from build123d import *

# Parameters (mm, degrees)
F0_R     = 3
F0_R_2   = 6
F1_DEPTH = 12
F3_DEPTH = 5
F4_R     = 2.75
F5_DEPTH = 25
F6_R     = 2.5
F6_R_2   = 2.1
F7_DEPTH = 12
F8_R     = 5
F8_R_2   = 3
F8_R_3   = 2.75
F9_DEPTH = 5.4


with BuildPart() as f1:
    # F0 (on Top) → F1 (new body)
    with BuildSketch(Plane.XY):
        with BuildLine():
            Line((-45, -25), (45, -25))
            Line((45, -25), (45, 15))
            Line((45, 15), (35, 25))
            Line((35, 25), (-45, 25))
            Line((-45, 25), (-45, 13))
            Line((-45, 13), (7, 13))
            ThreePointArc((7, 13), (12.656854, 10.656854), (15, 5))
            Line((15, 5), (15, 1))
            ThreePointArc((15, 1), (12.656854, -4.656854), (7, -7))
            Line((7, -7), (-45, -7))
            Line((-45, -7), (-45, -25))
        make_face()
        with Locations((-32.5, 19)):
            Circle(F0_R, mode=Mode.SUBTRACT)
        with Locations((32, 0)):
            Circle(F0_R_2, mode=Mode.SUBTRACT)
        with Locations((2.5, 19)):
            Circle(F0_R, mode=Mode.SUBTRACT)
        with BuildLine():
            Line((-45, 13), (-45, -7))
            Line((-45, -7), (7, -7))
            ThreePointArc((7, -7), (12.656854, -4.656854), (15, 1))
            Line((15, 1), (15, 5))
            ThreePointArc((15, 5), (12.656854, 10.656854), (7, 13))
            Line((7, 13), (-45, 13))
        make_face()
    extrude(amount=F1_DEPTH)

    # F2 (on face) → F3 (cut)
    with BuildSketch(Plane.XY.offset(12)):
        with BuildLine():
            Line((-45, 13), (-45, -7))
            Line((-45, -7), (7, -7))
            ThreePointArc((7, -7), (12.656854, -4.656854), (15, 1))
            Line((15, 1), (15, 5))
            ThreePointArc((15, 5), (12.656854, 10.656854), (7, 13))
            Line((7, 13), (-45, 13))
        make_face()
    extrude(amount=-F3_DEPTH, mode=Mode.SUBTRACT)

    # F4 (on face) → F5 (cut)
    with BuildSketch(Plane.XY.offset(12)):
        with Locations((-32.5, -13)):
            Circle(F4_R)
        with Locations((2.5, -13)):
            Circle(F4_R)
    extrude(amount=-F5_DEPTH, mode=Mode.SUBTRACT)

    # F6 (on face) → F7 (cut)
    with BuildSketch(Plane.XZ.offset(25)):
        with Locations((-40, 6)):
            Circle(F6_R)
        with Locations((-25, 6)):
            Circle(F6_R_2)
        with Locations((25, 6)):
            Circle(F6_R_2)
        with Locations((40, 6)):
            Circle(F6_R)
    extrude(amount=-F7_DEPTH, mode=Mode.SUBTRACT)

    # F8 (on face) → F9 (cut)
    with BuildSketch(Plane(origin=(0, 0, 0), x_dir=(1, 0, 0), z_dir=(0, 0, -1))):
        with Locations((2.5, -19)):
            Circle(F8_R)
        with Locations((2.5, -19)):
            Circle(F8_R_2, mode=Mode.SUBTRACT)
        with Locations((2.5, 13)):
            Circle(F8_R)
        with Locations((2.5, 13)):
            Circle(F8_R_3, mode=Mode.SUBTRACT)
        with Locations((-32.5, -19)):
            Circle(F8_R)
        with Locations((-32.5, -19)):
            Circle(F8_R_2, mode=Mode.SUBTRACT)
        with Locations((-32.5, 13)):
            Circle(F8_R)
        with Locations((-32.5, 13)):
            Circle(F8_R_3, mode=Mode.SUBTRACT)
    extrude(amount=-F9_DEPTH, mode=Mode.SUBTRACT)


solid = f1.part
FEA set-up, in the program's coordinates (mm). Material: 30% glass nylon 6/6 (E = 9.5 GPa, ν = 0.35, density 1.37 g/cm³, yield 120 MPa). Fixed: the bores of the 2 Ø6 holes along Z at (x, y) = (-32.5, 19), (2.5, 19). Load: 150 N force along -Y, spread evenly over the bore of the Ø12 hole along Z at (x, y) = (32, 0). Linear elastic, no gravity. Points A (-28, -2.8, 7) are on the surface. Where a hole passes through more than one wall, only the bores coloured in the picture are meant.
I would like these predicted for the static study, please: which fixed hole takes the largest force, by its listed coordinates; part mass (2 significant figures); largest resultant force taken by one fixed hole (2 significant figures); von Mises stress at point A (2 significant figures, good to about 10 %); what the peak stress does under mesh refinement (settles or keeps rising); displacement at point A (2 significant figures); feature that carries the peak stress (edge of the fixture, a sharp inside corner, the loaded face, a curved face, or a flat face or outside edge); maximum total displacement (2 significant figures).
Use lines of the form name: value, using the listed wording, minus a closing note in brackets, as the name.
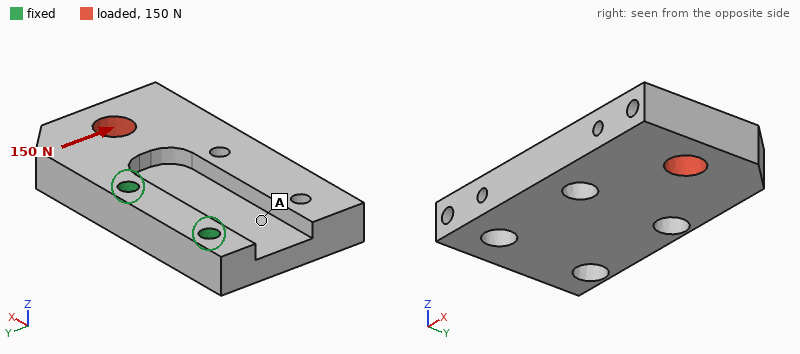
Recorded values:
which fixed hole takes the largest force, by its listed coordinates: (2.5, 19)
part mass: 59 g
largest resultant force taken by one fixed hole: 250 N
von Mises stress at point A: 1.1 MPa
what the peak stress does under mesh refinement: keeps rising
displacement at point A: 6.3 µm
feature that carries the peak stress: edge of the fixture
maximum total displacement: 34 µm
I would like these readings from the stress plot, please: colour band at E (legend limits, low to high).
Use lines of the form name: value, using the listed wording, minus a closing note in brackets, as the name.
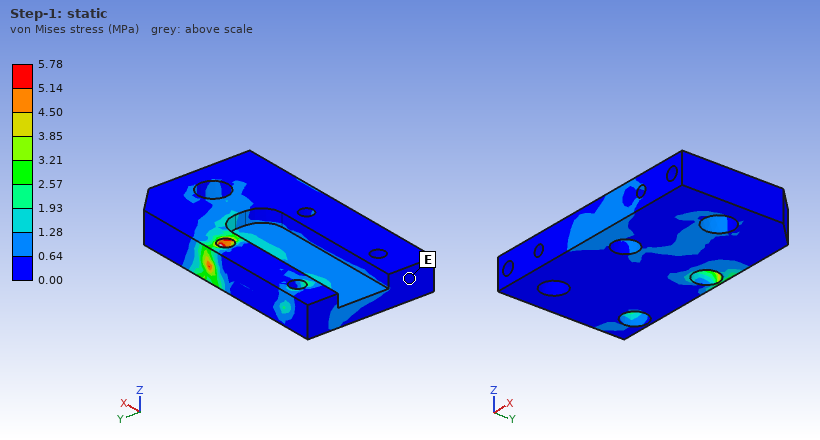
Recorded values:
colour band at E: 0.00 to 0.64 MPa
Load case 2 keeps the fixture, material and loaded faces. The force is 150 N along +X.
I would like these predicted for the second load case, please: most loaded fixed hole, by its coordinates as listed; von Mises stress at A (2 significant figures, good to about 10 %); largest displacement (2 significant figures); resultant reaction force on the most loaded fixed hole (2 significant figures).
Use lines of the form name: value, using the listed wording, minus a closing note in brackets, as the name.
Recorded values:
most loaded fixed hole, by its coordinates as listed: (2.5, 19)
von Mises stress at A: 0.63 MPa
largest displacement: 14 µm
resultant reaction force on the most loaded fixed hole: 120 N
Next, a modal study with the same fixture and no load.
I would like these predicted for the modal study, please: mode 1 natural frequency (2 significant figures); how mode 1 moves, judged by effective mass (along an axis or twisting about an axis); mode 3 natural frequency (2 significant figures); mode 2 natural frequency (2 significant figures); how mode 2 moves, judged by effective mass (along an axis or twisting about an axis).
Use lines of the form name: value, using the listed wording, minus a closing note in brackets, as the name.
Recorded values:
mode 1 natural frequency: 940 Hz
how mode 1 moves, judged by effective mass: along Z
mode 3 natural frequency: 2600 Hz
mode 2 natural frequency: 1600 Hz
how mode 2 moves, judged by effective mass: twisting about Y
